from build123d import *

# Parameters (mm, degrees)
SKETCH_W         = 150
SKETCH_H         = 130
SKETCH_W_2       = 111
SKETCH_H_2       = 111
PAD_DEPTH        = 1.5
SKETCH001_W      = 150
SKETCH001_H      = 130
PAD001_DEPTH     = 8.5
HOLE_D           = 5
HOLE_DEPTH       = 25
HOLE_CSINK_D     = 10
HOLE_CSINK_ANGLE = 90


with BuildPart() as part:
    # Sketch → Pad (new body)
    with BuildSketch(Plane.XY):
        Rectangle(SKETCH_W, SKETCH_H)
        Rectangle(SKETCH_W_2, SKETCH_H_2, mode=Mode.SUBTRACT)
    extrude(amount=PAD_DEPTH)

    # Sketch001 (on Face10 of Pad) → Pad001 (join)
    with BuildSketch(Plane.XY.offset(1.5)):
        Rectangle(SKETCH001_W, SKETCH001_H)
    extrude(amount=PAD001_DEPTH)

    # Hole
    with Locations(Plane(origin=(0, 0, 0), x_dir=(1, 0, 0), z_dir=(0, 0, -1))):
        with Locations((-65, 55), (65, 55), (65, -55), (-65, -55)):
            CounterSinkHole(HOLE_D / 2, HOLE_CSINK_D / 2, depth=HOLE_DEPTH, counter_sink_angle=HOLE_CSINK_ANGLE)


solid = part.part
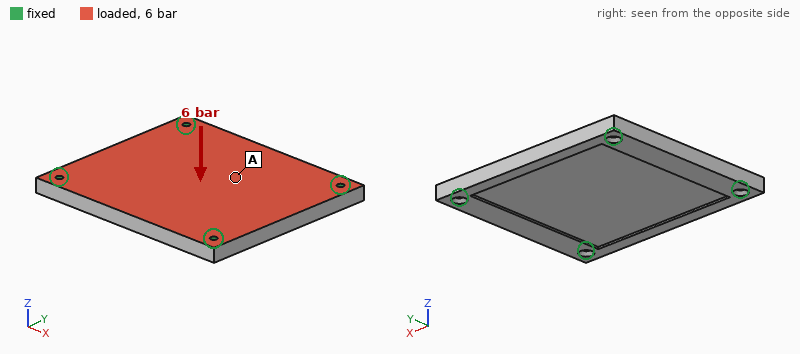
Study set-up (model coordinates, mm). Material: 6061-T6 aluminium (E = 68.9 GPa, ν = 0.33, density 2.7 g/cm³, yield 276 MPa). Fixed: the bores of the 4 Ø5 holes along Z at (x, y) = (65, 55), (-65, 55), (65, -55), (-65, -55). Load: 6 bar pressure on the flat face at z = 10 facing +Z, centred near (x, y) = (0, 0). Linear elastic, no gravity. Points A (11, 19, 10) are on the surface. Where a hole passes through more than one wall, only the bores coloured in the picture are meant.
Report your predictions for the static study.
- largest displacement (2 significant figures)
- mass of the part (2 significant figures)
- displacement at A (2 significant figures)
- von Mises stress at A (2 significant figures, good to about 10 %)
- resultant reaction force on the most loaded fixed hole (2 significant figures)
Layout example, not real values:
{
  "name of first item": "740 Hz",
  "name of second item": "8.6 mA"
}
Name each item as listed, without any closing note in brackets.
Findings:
{
  "largest displacement": "0.28 mm",
  "mass of the part": "470 g",
  "displacement at A": "0.26 mm",
  "von Mises stress at A": "40 MPa",
  "resultant reaction force on the most loaded fixed hole": "2.9 kN"
}
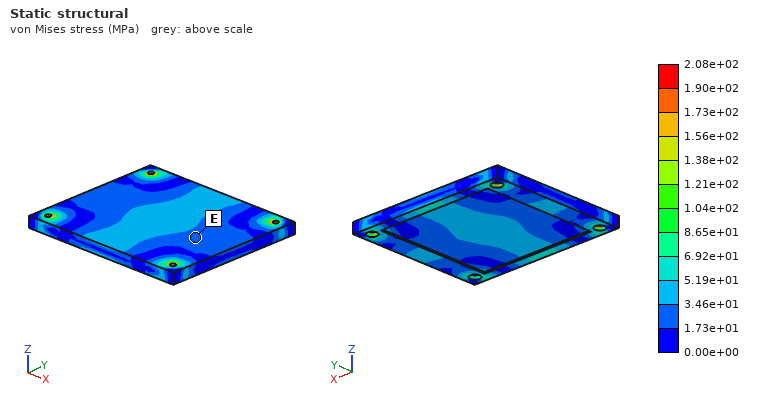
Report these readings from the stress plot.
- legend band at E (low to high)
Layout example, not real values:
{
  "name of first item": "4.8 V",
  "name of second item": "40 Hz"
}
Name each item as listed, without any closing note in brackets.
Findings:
{
  "legend band at E": "1.73e+01 to 3.46e+01 MPa"
}
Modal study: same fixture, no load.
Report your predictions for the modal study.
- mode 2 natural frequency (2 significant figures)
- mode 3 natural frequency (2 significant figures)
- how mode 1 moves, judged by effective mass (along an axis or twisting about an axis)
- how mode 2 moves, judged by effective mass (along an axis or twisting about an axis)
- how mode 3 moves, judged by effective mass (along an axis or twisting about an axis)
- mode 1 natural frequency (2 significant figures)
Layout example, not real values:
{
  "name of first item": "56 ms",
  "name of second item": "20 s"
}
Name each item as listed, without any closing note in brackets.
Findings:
{
  "mode 2 natural frequency": "2900 Hz",
  "mode 3 natural frequency": "3600 Hz",
  "how mode 1 moves, judged by effective mass": "along Z",
  "how mode 2 moves, judged by effective mass": "twisting about X",
  "how mode 3 moves, judged by effective mass": "twisting about Y",
  "mode 1 natural frequency": "1800 Hz"
}
